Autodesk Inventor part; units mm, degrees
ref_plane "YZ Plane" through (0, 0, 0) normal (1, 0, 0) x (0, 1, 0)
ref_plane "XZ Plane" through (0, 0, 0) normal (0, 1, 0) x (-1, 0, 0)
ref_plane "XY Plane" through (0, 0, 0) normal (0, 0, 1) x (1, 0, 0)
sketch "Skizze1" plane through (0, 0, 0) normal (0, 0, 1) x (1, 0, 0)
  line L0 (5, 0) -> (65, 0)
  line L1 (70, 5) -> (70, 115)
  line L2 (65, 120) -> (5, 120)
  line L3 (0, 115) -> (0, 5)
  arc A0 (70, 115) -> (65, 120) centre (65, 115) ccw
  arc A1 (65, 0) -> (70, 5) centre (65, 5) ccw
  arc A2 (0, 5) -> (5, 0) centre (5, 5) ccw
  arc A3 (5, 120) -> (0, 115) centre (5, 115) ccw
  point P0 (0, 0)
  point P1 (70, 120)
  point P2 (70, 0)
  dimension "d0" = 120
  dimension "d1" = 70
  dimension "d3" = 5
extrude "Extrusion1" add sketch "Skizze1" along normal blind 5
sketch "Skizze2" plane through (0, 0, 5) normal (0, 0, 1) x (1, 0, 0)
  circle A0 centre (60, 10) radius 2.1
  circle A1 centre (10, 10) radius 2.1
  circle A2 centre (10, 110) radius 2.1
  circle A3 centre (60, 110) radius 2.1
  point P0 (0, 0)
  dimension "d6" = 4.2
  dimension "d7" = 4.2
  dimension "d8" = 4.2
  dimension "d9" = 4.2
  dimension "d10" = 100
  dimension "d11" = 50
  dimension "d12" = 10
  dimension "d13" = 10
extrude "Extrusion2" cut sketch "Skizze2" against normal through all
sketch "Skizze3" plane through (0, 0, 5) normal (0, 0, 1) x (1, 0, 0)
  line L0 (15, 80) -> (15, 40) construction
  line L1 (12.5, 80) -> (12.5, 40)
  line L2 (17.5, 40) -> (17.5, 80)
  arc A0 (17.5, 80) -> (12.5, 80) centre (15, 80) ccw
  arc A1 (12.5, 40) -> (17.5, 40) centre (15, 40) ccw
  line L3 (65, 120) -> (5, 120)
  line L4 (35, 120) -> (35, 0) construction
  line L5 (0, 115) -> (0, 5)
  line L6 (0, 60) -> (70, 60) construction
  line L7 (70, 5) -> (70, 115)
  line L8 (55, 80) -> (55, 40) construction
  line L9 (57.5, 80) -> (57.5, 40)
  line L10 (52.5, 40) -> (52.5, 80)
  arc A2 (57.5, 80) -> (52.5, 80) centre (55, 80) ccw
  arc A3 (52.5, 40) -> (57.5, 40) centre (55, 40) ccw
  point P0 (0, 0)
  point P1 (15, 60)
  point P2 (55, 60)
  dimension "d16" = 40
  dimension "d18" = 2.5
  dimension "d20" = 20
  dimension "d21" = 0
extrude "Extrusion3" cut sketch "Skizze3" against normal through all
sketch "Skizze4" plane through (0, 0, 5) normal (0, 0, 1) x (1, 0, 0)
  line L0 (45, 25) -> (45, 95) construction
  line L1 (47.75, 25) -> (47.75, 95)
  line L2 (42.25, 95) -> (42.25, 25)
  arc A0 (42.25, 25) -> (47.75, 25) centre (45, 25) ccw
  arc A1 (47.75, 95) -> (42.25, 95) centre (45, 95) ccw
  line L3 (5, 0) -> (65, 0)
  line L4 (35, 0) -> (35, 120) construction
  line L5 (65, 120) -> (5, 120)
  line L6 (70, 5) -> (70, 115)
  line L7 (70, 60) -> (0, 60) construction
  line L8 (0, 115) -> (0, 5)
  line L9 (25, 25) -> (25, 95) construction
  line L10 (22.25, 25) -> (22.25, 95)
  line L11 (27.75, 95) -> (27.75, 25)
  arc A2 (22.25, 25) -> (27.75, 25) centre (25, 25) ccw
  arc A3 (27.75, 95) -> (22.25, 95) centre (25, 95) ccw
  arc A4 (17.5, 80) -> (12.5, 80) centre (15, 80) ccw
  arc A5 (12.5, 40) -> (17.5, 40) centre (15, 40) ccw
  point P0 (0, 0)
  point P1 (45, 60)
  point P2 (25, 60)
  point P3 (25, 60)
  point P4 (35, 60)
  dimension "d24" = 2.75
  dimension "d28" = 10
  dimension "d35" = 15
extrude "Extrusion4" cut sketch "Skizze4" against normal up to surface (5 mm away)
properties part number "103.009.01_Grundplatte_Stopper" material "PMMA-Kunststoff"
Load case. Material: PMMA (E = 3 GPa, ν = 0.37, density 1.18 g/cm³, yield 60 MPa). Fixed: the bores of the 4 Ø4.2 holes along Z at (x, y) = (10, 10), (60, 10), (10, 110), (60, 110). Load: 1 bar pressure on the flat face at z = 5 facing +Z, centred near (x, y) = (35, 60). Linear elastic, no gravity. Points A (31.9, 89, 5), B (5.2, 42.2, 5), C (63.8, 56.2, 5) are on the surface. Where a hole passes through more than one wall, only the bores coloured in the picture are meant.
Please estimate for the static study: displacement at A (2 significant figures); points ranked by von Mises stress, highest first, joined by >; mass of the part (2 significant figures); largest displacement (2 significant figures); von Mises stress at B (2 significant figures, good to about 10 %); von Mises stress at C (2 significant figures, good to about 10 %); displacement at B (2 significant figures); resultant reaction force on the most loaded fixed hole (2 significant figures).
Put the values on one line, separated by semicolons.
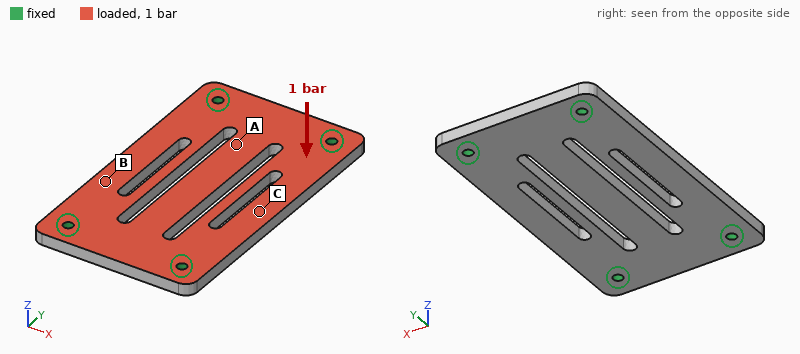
0.61 mm; C > B > A; 42 g; 1.2 mm; 5.9 MPa; 9.5 MPa; 0.63 mm; 180 N
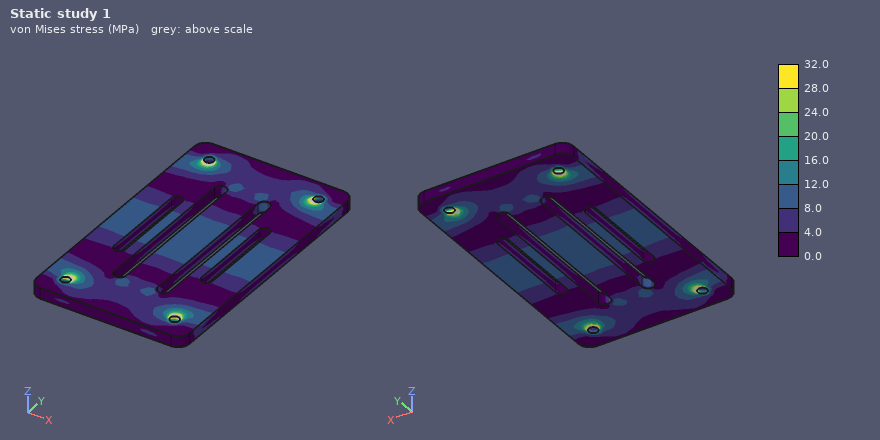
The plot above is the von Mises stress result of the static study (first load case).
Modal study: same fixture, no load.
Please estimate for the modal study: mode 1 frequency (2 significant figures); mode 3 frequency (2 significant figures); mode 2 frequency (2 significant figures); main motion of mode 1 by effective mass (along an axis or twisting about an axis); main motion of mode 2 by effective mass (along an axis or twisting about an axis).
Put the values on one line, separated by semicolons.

760 Hz; 970 Hz; 910 Hz; along Z; twisting about Y
